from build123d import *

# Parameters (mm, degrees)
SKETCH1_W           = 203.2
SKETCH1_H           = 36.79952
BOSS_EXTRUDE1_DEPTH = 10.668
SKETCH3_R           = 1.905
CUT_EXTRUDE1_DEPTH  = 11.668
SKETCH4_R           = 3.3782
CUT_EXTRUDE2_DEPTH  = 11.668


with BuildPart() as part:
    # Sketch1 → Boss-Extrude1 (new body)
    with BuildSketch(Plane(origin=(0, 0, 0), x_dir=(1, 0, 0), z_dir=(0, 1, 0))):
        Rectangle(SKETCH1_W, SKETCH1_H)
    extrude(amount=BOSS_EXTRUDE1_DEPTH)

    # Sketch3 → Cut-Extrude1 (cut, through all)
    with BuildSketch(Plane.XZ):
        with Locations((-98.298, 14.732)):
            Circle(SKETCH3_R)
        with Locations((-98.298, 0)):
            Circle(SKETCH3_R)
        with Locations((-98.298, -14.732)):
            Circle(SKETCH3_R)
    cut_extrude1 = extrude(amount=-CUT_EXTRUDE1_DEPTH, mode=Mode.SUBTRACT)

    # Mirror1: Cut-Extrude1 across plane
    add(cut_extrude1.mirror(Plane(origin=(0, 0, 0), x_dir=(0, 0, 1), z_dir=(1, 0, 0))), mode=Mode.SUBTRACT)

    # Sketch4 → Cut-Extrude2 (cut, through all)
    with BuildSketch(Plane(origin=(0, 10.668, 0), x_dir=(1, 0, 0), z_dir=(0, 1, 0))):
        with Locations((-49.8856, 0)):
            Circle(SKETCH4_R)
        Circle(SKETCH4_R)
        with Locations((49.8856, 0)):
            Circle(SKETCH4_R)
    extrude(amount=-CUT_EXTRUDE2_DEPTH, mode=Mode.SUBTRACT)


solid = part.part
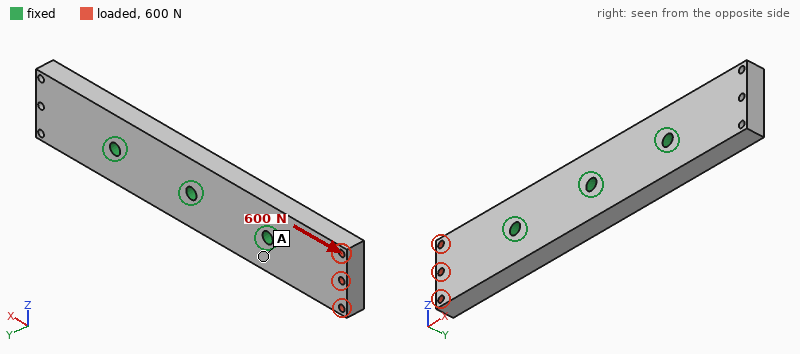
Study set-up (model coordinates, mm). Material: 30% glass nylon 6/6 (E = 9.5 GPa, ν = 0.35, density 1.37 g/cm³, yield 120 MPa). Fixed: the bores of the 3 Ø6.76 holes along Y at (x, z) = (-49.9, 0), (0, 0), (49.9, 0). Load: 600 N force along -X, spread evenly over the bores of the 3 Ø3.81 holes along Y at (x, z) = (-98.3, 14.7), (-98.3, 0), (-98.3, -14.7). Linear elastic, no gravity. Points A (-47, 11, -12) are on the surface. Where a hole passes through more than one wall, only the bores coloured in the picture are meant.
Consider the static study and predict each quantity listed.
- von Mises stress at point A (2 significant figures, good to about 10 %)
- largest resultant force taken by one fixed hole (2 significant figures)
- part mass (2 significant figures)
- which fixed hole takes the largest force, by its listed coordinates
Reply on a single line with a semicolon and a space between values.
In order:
0.84 MPa; 510 N; 110 g; (-49.9, 0)
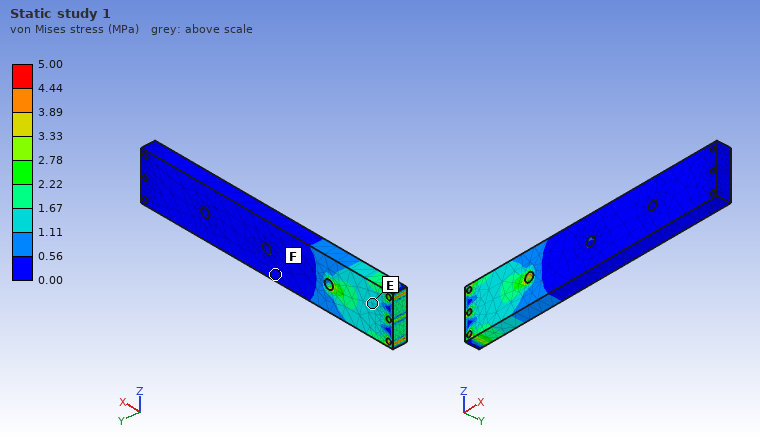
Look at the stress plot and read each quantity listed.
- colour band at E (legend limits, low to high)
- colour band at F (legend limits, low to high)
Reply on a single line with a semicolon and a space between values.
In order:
1.11 to 1.67 MPa; 0.00 to 0.56 MPa
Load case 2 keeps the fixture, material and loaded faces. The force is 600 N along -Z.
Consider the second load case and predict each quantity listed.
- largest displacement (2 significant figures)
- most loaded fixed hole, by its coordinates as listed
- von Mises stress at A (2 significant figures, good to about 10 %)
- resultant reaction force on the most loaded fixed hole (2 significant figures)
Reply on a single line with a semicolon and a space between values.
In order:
0.16 mm; (-49.9, 0); 6.4 MPa; 1.0 kN
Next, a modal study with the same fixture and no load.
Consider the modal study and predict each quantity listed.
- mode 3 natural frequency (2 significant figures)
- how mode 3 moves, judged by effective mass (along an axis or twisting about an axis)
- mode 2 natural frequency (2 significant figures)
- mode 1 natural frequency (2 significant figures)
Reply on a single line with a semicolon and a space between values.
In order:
3200 Hz; along Z; 1600 Hz; 1600 Hz
